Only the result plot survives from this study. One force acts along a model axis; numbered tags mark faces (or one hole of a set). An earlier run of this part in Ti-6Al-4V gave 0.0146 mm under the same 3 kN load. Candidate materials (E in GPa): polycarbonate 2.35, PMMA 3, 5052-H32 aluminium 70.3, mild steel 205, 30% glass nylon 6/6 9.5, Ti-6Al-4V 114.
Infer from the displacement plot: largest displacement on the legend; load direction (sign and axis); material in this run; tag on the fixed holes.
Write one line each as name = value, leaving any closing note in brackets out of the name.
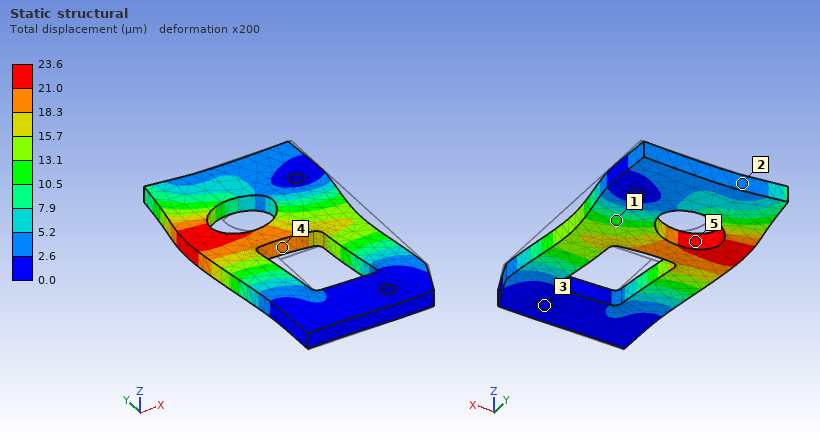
largest displacement on the legend = 23.6 µm
load direction = -X
material in this run = 5052-H32 aluminium
tag on the fixed holes = 3
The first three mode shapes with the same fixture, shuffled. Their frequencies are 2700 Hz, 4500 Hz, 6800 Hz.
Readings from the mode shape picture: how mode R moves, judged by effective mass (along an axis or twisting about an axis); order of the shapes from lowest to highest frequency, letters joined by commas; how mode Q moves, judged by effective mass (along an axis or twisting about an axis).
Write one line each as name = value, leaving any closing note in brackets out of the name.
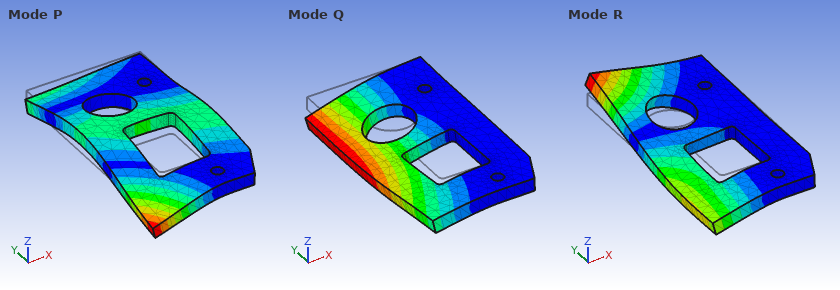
how mode R moves, judged by effective mass = twisting about X
order of the shapes from lowest to highest frequency, letters joined by commas = Q, R, P
how mode Q moves, judged by effective mass = along Z
